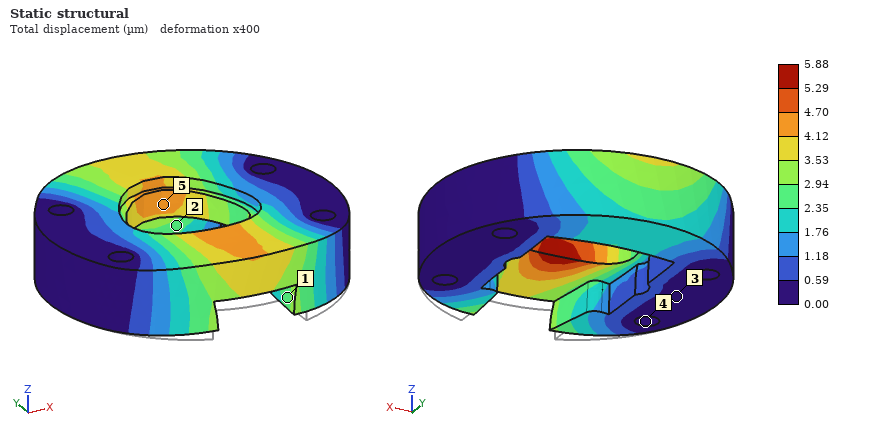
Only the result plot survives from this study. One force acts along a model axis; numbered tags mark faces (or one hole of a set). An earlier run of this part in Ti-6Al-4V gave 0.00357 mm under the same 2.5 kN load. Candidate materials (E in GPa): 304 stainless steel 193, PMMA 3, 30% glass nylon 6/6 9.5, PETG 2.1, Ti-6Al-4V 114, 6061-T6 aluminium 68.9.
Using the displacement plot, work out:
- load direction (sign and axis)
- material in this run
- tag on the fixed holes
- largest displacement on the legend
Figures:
+Y
6061-T6 aluminium
4
5.88 µm
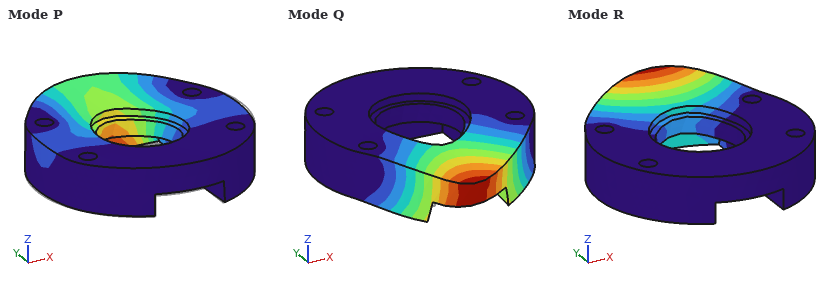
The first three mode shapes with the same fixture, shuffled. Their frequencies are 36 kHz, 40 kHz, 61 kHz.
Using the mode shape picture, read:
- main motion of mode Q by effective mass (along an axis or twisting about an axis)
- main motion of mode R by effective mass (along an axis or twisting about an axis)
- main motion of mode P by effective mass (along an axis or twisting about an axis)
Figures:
along Z
along Z
along Y
